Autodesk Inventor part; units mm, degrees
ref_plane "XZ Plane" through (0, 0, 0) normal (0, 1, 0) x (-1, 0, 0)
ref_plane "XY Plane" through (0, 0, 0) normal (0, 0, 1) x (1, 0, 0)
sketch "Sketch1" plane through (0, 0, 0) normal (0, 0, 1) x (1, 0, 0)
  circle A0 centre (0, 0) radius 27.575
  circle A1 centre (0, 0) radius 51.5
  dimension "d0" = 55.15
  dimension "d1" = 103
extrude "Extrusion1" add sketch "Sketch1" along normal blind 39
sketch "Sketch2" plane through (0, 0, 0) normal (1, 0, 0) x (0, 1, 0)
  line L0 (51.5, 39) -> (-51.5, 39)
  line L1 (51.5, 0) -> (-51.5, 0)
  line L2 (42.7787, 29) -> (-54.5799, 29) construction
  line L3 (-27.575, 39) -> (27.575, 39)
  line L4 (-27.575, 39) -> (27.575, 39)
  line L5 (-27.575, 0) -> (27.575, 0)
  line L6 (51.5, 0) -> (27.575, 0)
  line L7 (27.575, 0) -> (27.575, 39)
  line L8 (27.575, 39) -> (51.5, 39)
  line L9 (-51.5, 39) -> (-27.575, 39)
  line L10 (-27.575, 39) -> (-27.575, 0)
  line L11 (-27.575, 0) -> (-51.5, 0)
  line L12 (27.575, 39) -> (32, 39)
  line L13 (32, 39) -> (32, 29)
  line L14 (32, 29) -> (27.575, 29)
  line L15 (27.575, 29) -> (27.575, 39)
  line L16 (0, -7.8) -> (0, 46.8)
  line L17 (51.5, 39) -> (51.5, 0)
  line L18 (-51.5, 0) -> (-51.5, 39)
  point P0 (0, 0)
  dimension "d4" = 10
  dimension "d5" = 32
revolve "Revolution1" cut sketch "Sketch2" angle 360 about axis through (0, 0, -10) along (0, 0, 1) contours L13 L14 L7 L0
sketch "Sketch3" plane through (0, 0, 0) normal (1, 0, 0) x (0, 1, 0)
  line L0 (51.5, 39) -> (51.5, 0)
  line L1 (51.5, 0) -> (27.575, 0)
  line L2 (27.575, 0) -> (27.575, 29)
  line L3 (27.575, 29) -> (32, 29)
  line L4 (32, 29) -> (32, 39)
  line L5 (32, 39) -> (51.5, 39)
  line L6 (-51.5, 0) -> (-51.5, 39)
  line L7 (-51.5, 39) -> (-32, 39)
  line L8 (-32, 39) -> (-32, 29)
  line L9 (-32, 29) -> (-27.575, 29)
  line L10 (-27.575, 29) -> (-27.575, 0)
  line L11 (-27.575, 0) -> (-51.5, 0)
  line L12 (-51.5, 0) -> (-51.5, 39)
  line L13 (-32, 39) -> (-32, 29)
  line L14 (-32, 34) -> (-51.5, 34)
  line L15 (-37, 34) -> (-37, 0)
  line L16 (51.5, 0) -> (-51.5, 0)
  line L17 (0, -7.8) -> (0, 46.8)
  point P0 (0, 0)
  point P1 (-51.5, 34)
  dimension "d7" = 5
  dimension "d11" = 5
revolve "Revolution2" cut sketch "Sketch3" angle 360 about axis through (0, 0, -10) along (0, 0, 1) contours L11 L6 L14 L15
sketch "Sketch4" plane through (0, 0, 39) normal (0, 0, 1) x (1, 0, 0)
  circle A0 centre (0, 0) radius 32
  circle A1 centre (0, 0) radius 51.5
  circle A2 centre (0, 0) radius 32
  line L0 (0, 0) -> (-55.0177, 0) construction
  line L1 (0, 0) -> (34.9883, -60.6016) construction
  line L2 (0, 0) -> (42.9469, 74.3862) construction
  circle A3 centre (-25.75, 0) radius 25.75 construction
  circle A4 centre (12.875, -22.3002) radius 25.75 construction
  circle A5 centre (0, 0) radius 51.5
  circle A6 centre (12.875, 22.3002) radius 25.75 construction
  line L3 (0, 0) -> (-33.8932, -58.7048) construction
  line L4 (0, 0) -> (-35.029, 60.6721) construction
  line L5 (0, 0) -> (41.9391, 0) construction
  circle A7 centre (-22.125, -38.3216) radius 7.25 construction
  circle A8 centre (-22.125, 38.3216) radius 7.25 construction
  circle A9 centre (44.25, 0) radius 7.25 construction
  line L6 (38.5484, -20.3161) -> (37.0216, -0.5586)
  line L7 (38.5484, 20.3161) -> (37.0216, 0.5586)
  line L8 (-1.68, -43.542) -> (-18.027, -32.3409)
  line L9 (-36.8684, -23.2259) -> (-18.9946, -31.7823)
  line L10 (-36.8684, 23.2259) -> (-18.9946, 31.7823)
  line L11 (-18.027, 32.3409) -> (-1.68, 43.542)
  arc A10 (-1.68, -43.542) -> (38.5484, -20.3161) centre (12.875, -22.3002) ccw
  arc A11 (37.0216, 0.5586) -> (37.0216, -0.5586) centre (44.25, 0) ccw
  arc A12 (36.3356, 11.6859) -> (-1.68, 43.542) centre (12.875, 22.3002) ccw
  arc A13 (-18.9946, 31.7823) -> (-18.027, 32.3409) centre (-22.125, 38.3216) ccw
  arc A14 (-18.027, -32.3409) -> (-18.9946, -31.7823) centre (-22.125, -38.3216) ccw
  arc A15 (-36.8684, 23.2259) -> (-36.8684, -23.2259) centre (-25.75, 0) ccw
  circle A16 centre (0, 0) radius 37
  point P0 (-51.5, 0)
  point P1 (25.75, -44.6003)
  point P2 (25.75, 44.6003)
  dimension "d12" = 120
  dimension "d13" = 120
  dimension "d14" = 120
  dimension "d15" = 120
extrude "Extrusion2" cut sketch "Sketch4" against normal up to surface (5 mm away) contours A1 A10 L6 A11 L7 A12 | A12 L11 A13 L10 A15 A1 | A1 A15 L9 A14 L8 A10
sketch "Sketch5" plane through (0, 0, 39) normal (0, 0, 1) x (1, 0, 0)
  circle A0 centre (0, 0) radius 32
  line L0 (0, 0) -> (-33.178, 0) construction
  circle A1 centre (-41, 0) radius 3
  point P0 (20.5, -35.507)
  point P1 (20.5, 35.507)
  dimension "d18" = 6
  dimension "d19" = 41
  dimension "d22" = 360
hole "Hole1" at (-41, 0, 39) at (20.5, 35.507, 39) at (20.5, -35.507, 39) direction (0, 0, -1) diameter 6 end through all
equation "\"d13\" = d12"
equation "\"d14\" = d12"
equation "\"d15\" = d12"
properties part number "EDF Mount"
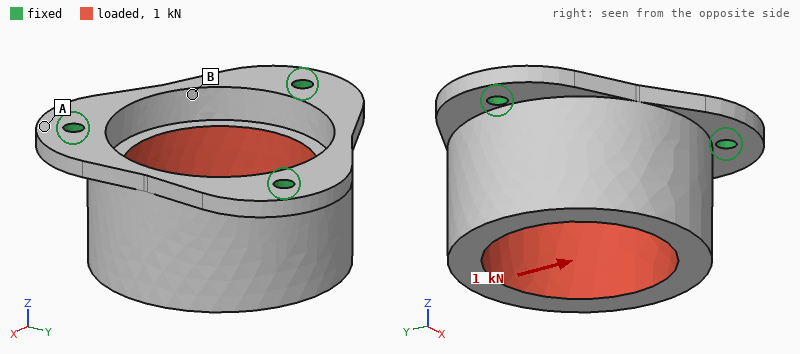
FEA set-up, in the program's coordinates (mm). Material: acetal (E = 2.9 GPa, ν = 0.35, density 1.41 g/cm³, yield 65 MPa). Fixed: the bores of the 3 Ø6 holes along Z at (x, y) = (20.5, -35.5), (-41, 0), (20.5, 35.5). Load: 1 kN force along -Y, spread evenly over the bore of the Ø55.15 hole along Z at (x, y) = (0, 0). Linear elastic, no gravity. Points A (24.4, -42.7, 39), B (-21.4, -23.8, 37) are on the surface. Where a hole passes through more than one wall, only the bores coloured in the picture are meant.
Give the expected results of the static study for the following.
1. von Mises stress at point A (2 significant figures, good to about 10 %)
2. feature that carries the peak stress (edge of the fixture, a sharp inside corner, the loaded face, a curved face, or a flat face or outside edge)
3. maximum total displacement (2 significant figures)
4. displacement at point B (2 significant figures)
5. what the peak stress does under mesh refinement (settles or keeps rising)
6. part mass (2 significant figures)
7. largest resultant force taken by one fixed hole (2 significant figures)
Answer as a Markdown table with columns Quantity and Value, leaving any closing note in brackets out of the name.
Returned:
| Quantity | Value |
|---|---|
| von Mises stress at point A | 3.2 MPa |
| feature that carries the peak stress | edge of the fixture |
| maximum total displacement | 0.16 mm |
| displacement at point B | 0.059 mm |
| what the peak stress does under mesh refinement | keeps rising |
| part mass | 110 g |
| largest resultant force taken by one fixed hole | 450 N |
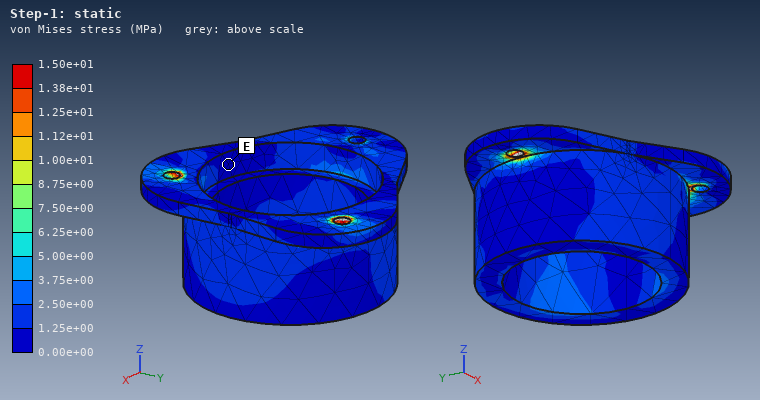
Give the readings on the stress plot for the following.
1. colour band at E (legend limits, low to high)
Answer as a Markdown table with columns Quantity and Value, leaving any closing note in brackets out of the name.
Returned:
| Quantity | Value |
|---|---|
| colour band at E | 0.00e+00 to 1.25e+00 MPa |
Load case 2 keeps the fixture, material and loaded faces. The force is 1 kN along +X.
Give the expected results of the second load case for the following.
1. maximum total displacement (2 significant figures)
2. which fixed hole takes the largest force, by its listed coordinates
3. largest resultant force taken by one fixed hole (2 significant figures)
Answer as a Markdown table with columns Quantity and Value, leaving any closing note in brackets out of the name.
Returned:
| Quantity | Value |
|---|---|
| maximum total displacement | 0.18 mm |
| which fixed hole takes the largest force, by its listed coordinates | (-41, 0) |
| largest resultant force taken by one fixed hole | 480 N |
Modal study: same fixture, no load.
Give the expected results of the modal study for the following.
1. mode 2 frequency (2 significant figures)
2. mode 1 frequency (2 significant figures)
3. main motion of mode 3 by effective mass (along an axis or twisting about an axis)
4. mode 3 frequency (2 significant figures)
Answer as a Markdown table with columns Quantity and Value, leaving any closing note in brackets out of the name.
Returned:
| Quantity | Value |
|---|---|
| mode 2 frequency | 1500 Hz |
| mode 1 frequency | 1500 Hz |
| main motion of mode 3 by effective mass | along Z |
| mode 3 frequency | 2400 Hz |
